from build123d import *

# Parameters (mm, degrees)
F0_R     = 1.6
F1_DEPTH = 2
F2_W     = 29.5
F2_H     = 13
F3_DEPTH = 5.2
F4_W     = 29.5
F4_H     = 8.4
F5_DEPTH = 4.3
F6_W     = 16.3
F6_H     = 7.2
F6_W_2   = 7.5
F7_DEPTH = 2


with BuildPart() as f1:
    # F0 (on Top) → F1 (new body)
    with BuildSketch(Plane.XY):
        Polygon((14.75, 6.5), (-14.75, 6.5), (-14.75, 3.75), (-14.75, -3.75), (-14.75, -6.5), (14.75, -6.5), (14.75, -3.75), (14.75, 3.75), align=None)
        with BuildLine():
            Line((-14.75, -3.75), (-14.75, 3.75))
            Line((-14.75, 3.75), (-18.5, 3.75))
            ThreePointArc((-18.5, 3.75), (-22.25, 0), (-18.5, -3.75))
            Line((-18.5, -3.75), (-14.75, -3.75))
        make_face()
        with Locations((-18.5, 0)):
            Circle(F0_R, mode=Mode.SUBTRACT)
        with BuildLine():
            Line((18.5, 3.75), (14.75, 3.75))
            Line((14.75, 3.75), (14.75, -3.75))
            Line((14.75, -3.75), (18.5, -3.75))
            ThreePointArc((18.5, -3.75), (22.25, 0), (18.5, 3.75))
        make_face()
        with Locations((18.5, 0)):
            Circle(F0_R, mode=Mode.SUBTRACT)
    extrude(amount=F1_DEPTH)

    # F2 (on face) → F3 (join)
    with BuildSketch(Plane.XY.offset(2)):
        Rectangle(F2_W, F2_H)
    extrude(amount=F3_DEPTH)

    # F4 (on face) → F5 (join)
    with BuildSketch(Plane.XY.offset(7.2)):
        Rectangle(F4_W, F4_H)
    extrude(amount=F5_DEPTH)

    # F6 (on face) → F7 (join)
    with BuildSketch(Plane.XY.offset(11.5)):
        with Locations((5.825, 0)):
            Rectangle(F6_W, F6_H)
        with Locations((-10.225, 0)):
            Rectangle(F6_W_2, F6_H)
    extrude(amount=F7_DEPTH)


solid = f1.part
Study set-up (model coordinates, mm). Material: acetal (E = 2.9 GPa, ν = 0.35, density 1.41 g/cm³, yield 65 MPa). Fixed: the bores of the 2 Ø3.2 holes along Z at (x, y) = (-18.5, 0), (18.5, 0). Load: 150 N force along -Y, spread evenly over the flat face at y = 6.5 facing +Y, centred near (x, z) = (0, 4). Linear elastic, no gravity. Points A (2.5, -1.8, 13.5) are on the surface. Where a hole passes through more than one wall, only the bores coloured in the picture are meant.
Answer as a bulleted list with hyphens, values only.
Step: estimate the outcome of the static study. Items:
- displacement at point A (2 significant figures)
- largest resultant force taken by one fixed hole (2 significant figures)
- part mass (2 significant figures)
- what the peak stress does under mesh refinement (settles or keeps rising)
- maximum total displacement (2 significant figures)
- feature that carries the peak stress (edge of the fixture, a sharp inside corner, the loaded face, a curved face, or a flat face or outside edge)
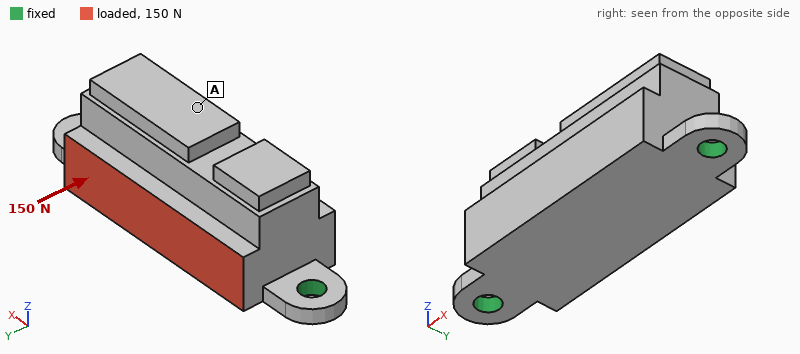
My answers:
- 0.32 mm
- 75 N
- 6.1 g
- keeps rising
- 0.33 mm
- edge of the fixture
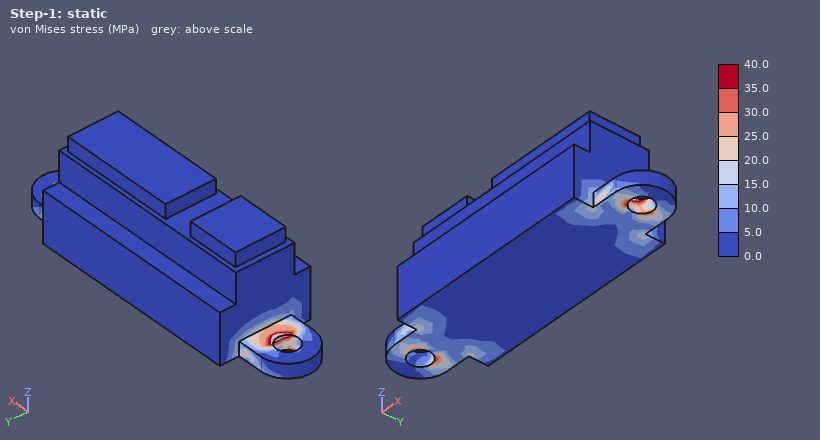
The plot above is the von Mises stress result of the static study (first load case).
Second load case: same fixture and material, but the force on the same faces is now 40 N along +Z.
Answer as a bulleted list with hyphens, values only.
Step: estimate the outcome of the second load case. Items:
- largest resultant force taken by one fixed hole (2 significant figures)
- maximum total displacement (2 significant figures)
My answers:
- 24 N
- 0.19 mm
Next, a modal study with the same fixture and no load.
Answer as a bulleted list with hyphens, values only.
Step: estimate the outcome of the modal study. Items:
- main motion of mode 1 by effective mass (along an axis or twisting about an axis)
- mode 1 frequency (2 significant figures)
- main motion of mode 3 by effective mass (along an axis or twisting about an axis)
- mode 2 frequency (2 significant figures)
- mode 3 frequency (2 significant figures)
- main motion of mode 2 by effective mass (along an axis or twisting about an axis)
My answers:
- along Y
- 1200 Hz
- along Y
- 3600 Hz
- 5800 Hz
- along Z
